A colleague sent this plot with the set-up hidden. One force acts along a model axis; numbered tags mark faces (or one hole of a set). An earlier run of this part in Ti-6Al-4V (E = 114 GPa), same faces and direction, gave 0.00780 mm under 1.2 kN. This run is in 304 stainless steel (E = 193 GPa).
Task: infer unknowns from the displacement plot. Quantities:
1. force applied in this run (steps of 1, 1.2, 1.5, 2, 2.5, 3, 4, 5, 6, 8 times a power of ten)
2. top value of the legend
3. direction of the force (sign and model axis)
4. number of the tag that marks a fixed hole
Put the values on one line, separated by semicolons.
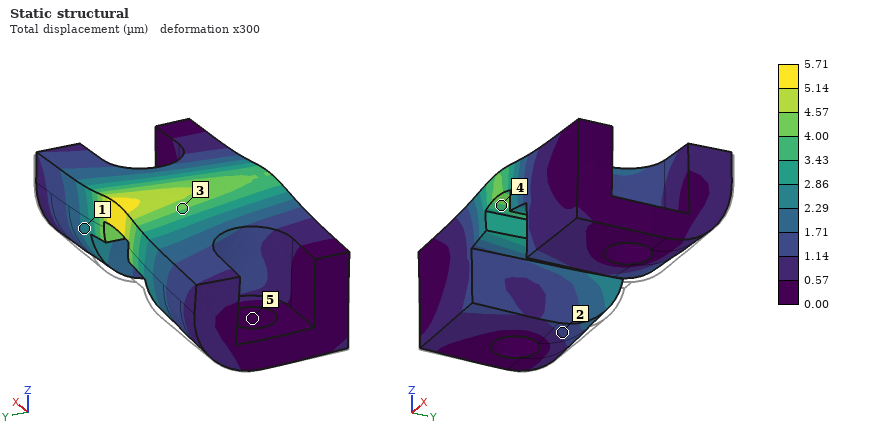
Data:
1.5 kN; 5.71 µm; +Z; 5
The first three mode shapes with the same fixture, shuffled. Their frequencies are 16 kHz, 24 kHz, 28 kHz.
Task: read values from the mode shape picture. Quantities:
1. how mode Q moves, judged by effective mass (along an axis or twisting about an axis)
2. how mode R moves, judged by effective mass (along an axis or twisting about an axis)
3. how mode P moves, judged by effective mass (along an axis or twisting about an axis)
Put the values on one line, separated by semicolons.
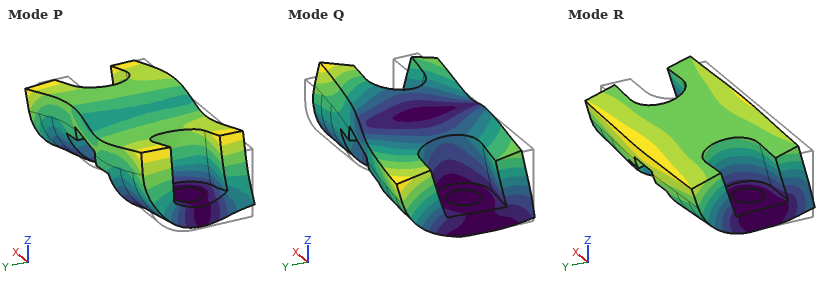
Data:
twisting about Z; along Y; along X
